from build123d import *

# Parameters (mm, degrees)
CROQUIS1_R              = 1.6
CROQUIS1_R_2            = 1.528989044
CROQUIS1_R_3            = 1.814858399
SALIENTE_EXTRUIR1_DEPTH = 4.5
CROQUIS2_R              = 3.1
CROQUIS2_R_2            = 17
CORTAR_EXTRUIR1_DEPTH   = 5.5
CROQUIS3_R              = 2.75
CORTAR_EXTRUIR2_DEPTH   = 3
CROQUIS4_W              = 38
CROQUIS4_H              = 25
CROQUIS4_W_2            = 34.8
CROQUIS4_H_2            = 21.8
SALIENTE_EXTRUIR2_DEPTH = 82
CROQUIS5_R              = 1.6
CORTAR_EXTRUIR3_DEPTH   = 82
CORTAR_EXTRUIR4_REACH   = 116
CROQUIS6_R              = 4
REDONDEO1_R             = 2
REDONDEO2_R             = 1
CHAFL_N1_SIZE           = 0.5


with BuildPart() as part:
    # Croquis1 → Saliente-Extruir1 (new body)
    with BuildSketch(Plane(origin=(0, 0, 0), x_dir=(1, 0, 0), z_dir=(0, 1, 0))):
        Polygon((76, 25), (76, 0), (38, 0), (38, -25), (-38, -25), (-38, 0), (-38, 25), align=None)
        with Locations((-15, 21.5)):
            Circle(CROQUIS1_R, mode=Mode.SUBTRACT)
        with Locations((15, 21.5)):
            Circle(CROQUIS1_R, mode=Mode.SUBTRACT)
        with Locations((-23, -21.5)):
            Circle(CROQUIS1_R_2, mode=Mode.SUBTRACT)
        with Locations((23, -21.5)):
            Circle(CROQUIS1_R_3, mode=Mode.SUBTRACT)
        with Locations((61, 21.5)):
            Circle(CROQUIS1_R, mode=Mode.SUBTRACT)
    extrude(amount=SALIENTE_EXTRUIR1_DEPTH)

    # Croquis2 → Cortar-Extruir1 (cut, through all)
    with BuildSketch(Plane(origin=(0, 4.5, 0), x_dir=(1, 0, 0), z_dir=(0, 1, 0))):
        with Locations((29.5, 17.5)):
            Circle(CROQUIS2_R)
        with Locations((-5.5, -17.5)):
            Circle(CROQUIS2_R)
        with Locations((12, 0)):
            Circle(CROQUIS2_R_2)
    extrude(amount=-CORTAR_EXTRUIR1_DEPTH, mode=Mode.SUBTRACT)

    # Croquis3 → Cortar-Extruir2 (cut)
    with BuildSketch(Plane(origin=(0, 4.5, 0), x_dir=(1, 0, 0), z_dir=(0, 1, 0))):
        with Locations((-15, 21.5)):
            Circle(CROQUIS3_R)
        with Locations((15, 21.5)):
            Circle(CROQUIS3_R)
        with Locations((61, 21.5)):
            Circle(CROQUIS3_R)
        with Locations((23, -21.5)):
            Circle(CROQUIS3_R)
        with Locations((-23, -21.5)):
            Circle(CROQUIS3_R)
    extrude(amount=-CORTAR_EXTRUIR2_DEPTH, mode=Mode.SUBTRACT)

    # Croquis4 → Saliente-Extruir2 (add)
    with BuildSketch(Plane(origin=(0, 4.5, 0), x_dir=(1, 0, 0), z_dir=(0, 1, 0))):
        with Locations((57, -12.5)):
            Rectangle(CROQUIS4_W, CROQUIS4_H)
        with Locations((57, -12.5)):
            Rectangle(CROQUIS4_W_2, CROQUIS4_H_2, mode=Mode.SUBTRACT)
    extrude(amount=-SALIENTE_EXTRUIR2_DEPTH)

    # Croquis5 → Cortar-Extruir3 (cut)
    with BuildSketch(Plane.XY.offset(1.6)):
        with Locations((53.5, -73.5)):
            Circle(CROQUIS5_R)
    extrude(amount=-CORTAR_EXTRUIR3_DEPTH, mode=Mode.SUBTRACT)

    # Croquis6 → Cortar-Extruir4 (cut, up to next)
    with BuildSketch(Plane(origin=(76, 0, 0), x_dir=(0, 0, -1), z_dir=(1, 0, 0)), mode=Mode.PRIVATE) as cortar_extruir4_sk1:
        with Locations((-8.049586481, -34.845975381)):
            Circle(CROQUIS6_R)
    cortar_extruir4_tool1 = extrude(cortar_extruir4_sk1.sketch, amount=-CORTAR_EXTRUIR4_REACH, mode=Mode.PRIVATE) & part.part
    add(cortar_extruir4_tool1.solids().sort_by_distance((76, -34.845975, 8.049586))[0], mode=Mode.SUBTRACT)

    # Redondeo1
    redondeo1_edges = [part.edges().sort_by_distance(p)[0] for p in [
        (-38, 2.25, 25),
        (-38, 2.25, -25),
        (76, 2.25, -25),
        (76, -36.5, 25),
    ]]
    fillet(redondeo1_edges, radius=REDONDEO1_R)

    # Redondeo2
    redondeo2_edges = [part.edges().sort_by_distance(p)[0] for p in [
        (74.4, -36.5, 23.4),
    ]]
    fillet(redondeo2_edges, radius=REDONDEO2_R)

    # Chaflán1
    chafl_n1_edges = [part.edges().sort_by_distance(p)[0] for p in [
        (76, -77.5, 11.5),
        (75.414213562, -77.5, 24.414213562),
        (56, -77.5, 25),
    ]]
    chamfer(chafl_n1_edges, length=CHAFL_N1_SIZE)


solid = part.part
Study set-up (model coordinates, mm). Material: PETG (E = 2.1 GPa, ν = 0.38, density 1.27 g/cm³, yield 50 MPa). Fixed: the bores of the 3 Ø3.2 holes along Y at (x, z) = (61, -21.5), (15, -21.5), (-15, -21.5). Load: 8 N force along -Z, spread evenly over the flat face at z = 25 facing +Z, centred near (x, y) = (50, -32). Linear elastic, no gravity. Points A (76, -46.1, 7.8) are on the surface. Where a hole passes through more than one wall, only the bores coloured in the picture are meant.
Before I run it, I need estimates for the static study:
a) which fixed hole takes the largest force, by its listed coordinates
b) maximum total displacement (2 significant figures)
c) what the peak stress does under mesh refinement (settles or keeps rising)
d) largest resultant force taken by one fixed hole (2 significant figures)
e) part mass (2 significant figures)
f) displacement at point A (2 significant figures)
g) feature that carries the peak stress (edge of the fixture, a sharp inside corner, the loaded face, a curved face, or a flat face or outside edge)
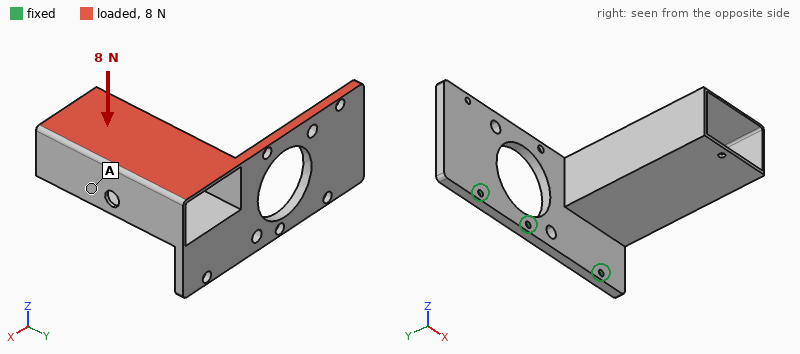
(61, -21.5)
1.6 mm
keeps rising
7.1 N
41 g
0.94 mm
edge of the fixture
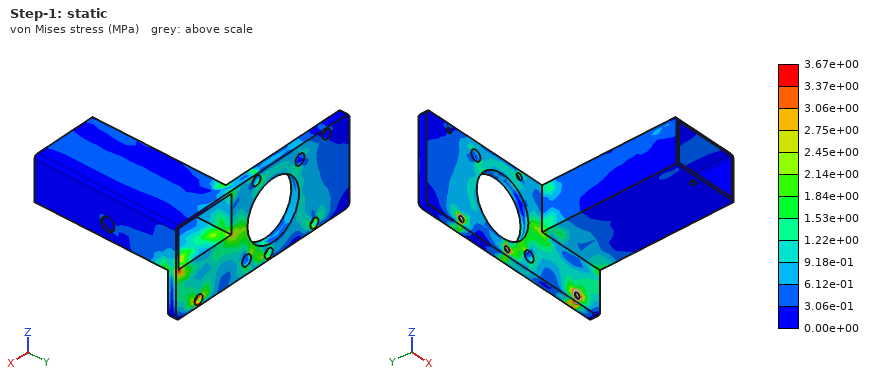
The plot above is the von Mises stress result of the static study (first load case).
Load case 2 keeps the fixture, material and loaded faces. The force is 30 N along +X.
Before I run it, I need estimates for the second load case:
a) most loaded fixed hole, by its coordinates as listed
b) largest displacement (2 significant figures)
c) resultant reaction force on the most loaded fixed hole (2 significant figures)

(61, -21.5)
1.8 mm
42 N
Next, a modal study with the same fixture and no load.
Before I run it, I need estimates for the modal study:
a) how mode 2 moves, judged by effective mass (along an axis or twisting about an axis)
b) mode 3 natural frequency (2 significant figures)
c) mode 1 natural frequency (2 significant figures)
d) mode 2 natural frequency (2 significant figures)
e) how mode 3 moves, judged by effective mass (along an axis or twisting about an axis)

along X
310 Hz
81 Hz
170 Hz
along Y
